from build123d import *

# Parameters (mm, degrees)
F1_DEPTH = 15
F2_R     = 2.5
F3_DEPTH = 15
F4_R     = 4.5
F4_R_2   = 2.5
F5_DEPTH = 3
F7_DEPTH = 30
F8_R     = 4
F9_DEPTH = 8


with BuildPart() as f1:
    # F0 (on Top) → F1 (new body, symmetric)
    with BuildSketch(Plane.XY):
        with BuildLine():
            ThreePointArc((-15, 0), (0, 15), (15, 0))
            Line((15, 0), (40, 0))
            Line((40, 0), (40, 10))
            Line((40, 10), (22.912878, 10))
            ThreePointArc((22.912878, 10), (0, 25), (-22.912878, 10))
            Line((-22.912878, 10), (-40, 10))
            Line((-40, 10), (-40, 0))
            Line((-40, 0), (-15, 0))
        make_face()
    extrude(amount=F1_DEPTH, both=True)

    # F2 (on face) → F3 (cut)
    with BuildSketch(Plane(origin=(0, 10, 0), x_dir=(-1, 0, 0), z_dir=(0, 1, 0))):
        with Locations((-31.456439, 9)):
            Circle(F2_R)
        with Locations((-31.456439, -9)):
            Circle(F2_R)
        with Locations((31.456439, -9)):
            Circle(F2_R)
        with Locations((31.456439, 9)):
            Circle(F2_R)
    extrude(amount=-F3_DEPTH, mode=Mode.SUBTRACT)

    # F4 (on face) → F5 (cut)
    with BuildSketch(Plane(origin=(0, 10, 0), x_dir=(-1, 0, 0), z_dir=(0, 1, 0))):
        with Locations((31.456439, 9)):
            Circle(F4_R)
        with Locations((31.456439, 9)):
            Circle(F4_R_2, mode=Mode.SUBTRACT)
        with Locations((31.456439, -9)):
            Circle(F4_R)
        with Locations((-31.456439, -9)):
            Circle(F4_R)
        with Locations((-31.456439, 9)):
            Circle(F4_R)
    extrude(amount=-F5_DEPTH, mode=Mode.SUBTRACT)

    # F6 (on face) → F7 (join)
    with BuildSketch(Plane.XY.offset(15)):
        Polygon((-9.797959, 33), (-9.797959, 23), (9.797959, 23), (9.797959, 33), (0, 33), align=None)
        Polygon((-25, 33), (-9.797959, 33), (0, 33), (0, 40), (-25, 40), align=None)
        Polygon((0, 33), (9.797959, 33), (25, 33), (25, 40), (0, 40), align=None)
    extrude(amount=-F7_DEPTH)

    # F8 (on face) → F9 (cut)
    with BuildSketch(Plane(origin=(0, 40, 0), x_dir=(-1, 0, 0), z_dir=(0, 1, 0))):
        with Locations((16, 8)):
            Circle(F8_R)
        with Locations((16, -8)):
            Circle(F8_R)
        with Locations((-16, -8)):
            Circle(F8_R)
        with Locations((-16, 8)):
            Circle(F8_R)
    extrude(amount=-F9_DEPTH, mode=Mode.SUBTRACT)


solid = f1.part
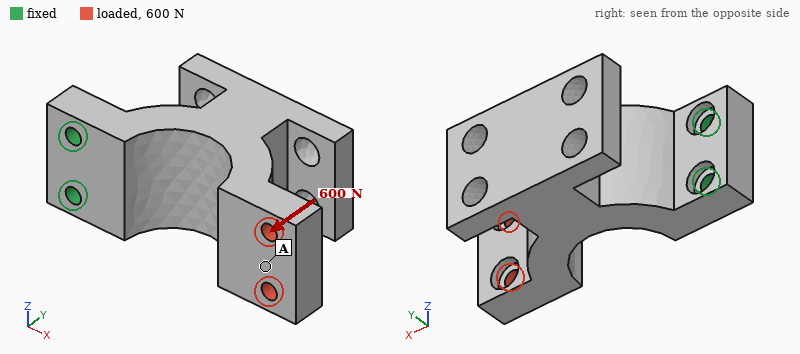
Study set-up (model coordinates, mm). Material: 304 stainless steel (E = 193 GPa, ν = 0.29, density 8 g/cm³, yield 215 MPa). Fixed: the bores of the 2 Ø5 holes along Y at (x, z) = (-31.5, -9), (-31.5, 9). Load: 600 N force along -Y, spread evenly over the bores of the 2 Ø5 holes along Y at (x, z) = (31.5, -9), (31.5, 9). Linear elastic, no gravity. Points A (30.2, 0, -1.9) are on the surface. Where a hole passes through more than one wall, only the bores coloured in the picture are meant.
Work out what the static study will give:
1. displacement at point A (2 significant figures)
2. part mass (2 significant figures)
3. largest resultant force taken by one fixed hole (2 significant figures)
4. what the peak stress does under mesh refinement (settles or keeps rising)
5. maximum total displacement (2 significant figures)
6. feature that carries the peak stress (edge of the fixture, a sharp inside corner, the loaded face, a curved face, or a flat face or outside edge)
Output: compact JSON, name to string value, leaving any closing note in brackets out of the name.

{"displacement at point A": "0.13 mm", "part mass": "330 g", "largest resultant force taken by one fixed hole": "300 N", "what the peak stress does under mesh refinement": "keeps rising", "maximum total displacement": "0.16 mm", "feature that carries the peak stress": "edge of the fixture"}
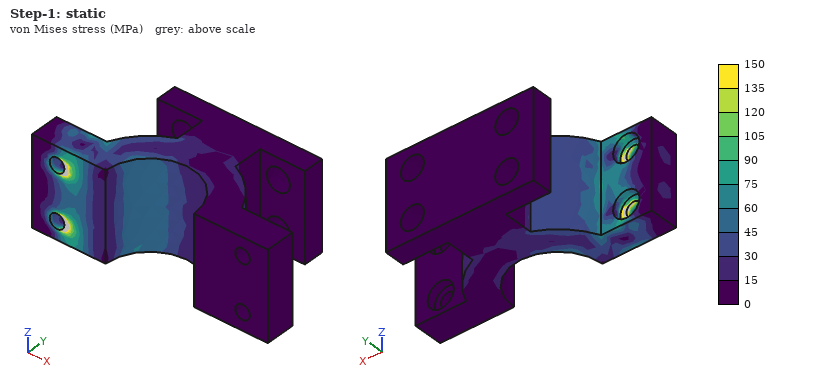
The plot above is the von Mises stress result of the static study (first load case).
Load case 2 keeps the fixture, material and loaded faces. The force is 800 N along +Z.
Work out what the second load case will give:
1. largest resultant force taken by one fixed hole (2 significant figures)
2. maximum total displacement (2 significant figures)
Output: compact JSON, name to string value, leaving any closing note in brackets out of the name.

{"largest resultant force taken by one fixed hole": "2.4 kN", "maximum total displacement": "63 µm"}
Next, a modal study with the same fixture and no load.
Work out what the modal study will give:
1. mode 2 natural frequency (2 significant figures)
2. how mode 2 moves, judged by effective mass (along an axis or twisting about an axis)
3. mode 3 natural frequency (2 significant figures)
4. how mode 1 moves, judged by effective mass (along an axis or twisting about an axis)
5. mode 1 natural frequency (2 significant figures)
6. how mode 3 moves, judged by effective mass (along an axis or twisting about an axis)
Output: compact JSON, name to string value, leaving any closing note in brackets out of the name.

{"mode 2 natural frequency": "2400 Hz", "how mode 2 moves, judged by effective mass": "along Z", "mode 3 natural frequency": "3300 Hz", "how mode 1 moves, judged by effective mass": "along Y", "mode 1 natural frequency": "1000 Hz", "how mode 3 moves, judged by effective mass": "along Z"}
